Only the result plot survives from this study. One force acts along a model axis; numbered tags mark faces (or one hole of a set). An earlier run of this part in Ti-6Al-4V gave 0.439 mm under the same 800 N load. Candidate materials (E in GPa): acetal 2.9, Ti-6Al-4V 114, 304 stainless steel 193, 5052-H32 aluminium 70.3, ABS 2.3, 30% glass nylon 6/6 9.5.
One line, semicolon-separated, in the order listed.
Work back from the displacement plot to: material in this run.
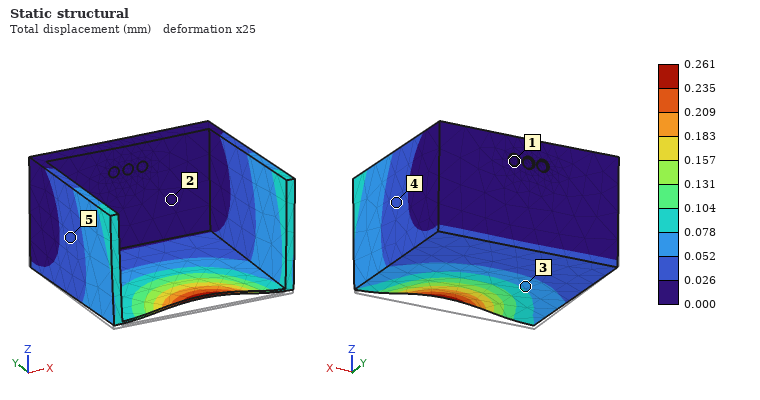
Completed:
304 stainless steel
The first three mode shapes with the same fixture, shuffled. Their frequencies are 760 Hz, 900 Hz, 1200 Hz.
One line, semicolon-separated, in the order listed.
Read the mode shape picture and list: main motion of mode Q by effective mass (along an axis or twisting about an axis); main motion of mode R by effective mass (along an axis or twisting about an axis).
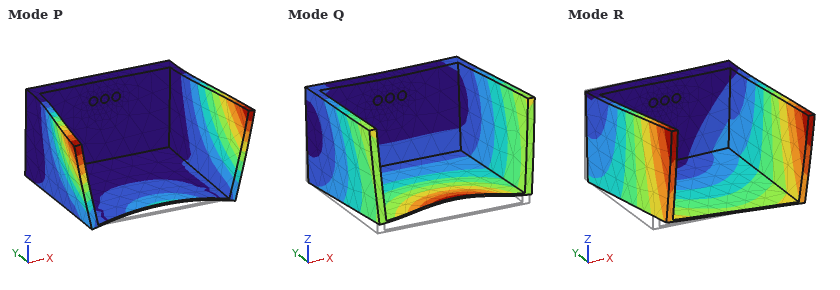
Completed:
along Z; along X
